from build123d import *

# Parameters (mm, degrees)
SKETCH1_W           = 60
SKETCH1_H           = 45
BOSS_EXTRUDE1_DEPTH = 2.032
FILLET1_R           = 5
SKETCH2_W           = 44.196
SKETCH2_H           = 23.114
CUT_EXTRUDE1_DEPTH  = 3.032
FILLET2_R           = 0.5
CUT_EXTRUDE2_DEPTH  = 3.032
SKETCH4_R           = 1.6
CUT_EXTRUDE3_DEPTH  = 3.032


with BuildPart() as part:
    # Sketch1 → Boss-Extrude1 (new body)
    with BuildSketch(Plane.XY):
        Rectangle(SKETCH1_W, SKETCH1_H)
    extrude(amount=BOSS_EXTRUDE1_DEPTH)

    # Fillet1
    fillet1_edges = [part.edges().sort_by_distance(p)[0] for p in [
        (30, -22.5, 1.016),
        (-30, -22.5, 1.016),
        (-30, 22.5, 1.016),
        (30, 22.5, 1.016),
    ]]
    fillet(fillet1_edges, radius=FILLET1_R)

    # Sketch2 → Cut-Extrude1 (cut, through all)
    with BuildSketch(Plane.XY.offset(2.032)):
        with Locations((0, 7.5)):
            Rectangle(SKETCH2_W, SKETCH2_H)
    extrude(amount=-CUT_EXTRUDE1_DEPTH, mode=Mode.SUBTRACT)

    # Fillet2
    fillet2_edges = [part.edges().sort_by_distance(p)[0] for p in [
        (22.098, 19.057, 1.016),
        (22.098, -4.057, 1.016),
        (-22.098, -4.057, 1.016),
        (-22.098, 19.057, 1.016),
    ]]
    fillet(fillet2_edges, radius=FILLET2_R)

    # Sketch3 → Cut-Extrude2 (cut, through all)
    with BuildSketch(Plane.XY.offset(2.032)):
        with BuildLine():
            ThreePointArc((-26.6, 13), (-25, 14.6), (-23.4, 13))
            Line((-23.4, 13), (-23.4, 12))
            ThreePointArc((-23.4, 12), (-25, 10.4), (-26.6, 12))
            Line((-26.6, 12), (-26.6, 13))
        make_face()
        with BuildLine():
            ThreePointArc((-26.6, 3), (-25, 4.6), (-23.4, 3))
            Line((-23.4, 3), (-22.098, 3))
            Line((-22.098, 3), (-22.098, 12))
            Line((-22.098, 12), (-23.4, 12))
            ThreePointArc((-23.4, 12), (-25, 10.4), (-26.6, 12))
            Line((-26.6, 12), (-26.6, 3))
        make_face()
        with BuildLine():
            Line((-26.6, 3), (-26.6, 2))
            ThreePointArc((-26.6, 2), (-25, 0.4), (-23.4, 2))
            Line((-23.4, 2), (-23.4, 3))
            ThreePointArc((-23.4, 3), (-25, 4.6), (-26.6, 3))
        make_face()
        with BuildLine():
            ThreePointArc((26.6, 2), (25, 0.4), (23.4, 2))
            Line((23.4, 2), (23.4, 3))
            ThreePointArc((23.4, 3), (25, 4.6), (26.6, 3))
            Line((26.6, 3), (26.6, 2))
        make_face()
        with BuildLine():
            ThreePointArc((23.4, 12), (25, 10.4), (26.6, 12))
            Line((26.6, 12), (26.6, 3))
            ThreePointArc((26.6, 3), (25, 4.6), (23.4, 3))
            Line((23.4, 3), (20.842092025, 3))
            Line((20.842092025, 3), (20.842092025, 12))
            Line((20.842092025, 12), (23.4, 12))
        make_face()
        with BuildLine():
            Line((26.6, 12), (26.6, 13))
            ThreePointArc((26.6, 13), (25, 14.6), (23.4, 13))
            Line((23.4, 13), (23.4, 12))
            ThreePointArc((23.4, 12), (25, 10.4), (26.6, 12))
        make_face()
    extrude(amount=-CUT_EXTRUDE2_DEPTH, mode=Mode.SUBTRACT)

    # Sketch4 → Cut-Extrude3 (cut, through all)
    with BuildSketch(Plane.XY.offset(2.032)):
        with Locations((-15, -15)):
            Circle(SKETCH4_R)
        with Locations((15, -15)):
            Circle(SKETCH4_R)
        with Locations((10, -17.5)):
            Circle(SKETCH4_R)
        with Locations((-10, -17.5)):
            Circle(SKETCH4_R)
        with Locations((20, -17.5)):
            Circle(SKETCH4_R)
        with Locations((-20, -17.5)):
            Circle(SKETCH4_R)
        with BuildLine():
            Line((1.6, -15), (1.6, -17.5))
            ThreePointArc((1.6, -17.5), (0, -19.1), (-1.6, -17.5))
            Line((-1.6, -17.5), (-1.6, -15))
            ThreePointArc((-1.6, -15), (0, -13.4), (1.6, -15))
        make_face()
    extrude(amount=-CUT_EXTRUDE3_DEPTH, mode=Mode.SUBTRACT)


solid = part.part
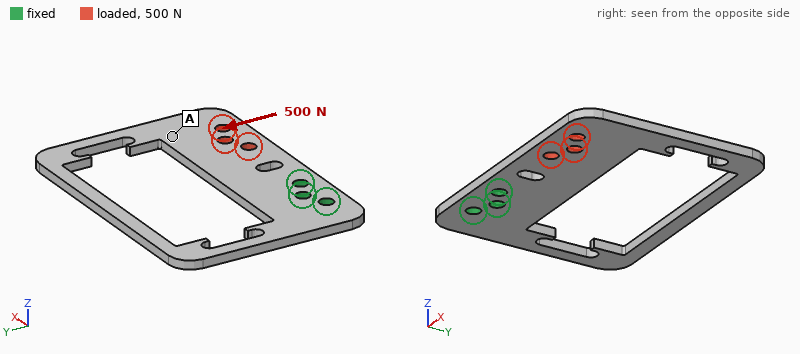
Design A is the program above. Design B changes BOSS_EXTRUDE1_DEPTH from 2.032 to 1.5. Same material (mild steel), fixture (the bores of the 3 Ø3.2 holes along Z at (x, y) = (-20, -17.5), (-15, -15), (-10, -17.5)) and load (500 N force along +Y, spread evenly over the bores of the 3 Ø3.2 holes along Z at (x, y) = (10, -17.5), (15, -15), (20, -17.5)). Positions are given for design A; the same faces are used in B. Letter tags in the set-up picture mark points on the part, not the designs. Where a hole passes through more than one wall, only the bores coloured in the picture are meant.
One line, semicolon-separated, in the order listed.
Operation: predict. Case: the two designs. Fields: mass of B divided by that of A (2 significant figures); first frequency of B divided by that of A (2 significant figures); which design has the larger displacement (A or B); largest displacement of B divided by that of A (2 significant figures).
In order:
0.74; 0.75; B; 1.4
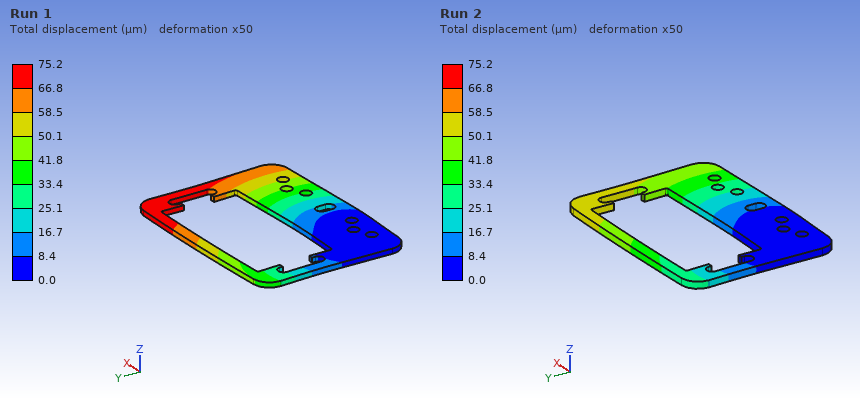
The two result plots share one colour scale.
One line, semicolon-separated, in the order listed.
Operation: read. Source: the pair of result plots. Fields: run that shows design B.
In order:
Run 1
